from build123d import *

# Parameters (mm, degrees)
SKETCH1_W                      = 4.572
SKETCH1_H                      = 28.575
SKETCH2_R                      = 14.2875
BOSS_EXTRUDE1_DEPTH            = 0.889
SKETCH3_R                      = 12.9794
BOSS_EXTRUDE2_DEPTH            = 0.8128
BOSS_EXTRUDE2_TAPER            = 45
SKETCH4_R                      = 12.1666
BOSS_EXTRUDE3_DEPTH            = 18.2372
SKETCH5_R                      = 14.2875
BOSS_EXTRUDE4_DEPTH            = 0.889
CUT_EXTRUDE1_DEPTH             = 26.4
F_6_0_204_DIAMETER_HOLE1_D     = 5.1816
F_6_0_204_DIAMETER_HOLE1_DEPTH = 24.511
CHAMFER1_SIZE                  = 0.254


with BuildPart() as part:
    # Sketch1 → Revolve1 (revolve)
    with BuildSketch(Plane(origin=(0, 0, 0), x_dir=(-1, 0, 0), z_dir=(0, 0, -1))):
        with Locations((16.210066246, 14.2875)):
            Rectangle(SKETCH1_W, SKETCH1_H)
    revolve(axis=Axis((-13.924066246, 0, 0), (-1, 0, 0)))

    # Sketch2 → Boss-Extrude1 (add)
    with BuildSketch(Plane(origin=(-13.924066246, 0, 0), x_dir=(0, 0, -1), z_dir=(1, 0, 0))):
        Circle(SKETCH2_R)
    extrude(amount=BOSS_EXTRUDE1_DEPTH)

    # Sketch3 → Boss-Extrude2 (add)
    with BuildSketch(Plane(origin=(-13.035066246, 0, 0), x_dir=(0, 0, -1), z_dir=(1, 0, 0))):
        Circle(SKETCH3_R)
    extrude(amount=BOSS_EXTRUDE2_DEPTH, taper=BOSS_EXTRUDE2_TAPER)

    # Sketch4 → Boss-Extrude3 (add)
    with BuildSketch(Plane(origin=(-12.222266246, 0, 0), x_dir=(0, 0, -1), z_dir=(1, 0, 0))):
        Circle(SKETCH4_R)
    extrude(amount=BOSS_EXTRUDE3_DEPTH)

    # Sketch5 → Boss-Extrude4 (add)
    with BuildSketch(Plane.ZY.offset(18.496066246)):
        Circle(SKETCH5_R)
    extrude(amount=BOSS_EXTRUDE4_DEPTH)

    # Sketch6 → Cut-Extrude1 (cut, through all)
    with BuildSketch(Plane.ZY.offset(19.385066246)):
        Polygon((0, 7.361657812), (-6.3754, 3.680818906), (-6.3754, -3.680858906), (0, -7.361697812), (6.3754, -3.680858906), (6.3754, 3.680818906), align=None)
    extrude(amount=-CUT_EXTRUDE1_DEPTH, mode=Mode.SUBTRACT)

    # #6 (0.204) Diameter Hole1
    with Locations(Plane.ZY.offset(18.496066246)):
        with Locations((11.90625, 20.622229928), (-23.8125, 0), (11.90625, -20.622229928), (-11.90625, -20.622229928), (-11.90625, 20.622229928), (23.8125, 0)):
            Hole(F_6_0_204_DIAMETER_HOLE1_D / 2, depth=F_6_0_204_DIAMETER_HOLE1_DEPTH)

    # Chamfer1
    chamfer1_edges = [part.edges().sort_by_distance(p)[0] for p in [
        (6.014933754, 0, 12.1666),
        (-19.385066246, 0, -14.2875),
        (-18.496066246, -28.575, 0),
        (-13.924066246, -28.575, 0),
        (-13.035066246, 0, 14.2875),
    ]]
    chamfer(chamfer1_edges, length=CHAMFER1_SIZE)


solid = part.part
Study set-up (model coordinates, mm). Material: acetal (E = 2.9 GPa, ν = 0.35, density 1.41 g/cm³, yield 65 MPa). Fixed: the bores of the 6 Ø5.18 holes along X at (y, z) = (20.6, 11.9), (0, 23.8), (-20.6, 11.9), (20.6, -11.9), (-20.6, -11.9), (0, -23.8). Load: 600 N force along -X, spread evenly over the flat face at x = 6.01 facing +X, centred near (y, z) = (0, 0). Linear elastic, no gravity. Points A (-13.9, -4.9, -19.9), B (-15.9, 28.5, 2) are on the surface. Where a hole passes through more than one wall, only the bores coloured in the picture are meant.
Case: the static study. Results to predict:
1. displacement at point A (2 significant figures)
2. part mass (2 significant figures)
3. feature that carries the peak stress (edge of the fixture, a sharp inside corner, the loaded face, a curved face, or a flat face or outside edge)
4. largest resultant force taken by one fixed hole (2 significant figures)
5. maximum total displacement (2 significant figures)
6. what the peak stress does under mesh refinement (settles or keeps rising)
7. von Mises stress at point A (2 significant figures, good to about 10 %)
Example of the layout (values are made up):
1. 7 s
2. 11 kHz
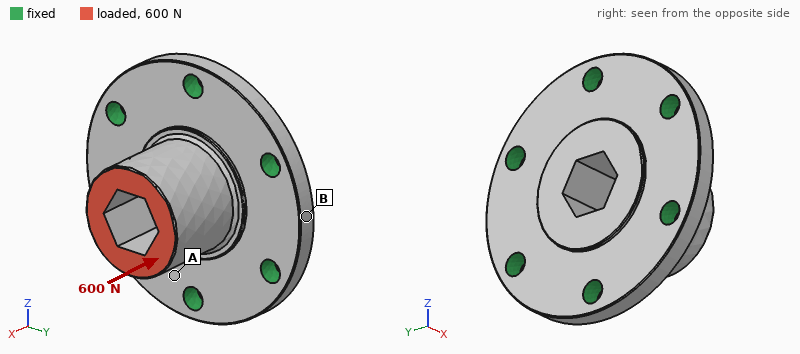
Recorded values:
1. 12 µm
2. 25 g
3. edge of the fixture
4. 110 N
5. 64 µm
6. keeps rising
7. 2.3 MPa
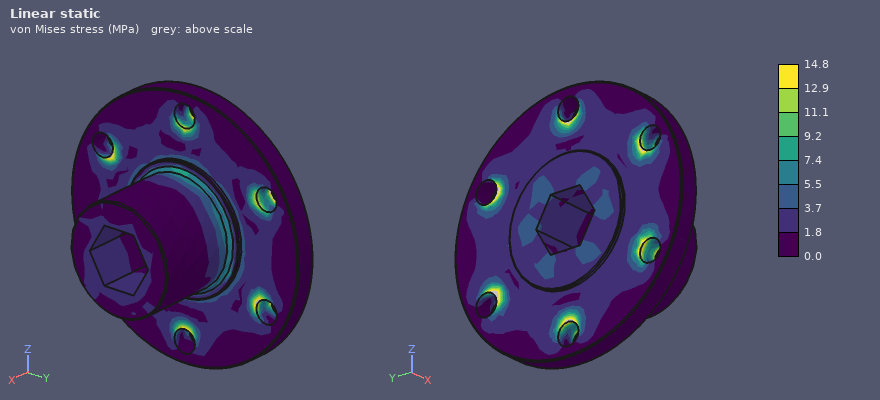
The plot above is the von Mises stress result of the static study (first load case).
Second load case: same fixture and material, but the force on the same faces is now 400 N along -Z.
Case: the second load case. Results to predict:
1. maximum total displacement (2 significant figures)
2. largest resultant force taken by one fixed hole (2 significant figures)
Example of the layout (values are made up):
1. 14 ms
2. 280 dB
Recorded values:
1. 0.18 mm
2. 190 N
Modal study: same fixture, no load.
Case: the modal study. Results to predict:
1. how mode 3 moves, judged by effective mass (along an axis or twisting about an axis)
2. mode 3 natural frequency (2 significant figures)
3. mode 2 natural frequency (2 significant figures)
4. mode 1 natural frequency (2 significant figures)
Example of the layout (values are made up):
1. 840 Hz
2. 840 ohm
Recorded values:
1. along X
2. 4400 Hz
3. 4100 Hz
4. 4100 Hz
